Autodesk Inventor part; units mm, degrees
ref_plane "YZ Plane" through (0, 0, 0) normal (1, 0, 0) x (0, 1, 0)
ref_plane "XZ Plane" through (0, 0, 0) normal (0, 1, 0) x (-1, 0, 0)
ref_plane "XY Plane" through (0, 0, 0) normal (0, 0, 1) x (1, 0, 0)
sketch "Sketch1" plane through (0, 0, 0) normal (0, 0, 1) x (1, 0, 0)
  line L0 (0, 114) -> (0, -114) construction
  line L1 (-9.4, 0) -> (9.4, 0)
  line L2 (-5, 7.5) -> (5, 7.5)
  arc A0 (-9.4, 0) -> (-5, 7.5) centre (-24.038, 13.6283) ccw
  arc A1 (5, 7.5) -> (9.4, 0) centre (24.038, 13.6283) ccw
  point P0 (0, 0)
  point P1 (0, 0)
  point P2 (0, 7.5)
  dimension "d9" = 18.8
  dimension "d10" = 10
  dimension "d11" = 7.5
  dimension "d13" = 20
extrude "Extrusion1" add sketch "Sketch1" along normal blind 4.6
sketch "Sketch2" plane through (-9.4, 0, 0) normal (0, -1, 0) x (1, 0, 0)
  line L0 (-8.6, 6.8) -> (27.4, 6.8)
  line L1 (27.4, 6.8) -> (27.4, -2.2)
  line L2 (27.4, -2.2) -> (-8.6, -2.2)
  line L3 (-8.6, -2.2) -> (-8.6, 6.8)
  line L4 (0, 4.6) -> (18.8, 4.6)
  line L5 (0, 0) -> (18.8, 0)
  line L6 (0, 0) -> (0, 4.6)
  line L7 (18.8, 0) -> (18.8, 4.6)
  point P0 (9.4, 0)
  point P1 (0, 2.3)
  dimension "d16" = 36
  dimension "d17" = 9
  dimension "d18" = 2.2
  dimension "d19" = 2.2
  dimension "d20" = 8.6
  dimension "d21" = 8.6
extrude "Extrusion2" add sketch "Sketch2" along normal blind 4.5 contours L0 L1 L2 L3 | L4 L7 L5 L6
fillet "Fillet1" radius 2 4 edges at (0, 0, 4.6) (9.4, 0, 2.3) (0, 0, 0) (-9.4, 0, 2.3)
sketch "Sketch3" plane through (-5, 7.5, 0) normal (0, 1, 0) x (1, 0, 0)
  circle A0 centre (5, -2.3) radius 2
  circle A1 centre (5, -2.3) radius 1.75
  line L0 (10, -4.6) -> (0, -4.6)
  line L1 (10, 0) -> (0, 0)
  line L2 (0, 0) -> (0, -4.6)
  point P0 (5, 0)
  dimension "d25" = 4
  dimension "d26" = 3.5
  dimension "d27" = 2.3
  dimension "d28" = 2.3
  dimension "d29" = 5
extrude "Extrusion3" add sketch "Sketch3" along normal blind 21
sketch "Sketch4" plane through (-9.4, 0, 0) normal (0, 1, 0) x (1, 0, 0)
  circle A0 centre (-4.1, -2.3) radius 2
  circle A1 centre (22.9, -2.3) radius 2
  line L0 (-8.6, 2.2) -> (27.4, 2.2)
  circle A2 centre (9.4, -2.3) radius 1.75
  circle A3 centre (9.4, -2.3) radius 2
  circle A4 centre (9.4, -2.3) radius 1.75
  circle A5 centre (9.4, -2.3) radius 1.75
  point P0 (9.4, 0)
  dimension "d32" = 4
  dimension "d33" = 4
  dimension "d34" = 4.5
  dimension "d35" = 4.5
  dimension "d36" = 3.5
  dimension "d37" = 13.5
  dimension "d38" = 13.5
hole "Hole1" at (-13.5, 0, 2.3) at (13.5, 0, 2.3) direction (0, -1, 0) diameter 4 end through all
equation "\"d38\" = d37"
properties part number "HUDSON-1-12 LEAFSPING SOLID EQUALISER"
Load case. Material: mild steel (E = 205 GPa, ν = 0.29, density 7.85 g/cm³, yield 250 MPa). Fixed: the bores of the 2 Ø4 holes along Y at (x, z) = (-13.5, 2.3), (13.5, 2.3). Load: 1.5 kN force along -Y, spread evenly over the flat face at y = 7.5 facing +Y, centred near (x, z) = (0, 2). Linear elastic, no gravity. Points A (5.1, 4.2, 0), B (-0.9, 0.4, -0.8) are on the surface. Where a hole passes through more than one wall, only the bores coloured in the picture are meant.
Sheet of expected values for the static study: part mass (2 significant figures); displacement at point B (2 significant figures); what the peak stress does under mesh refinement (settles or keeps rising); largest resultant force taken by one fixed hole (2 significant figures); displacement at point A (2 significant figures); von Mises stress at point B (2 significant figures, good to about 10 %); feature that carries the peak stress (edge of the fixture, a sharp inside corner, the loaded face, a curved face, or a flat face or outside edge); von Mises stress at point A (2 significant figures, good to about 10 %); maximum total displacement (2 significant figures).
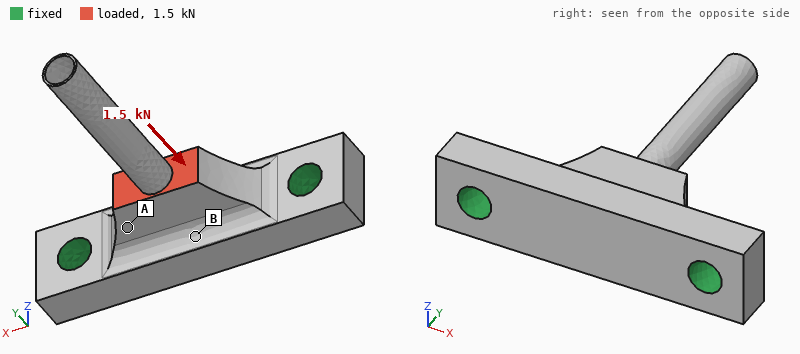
15 g
3.8 µm
keeps rising
830 N
3.5 µm
16 MPa
edge of the fixture
43 MPa
4.4 µm
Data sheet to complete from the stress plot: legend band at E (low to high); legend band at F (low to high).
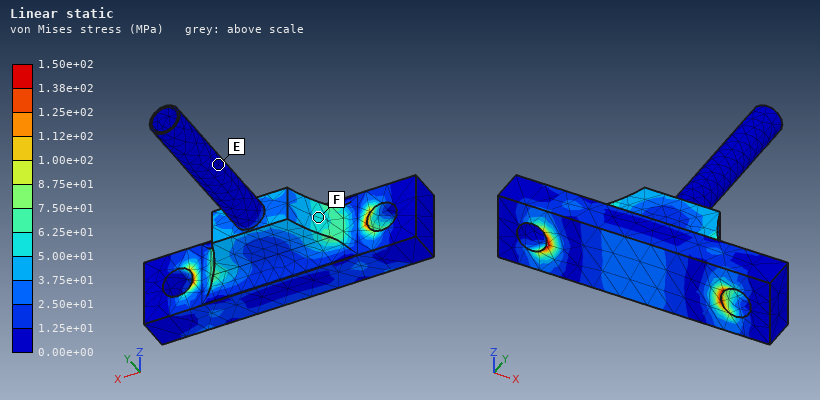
0.00e+00 to 1.25e+01 MPa
5.00e+01 to 6.25e+01 MPa
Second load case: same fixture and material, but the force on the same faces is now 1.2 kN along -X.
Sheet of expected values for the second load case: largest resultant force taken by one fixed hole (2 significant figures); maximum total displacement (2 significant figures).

820 N
7.7 µm
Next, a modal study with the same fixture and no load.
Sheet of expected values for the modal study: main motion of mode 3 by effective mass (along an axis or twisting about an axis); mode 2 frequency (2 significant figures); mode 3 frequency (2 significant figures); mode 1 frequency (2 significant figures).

along Z
7800 Hz
23 kHz
7200 Hz
